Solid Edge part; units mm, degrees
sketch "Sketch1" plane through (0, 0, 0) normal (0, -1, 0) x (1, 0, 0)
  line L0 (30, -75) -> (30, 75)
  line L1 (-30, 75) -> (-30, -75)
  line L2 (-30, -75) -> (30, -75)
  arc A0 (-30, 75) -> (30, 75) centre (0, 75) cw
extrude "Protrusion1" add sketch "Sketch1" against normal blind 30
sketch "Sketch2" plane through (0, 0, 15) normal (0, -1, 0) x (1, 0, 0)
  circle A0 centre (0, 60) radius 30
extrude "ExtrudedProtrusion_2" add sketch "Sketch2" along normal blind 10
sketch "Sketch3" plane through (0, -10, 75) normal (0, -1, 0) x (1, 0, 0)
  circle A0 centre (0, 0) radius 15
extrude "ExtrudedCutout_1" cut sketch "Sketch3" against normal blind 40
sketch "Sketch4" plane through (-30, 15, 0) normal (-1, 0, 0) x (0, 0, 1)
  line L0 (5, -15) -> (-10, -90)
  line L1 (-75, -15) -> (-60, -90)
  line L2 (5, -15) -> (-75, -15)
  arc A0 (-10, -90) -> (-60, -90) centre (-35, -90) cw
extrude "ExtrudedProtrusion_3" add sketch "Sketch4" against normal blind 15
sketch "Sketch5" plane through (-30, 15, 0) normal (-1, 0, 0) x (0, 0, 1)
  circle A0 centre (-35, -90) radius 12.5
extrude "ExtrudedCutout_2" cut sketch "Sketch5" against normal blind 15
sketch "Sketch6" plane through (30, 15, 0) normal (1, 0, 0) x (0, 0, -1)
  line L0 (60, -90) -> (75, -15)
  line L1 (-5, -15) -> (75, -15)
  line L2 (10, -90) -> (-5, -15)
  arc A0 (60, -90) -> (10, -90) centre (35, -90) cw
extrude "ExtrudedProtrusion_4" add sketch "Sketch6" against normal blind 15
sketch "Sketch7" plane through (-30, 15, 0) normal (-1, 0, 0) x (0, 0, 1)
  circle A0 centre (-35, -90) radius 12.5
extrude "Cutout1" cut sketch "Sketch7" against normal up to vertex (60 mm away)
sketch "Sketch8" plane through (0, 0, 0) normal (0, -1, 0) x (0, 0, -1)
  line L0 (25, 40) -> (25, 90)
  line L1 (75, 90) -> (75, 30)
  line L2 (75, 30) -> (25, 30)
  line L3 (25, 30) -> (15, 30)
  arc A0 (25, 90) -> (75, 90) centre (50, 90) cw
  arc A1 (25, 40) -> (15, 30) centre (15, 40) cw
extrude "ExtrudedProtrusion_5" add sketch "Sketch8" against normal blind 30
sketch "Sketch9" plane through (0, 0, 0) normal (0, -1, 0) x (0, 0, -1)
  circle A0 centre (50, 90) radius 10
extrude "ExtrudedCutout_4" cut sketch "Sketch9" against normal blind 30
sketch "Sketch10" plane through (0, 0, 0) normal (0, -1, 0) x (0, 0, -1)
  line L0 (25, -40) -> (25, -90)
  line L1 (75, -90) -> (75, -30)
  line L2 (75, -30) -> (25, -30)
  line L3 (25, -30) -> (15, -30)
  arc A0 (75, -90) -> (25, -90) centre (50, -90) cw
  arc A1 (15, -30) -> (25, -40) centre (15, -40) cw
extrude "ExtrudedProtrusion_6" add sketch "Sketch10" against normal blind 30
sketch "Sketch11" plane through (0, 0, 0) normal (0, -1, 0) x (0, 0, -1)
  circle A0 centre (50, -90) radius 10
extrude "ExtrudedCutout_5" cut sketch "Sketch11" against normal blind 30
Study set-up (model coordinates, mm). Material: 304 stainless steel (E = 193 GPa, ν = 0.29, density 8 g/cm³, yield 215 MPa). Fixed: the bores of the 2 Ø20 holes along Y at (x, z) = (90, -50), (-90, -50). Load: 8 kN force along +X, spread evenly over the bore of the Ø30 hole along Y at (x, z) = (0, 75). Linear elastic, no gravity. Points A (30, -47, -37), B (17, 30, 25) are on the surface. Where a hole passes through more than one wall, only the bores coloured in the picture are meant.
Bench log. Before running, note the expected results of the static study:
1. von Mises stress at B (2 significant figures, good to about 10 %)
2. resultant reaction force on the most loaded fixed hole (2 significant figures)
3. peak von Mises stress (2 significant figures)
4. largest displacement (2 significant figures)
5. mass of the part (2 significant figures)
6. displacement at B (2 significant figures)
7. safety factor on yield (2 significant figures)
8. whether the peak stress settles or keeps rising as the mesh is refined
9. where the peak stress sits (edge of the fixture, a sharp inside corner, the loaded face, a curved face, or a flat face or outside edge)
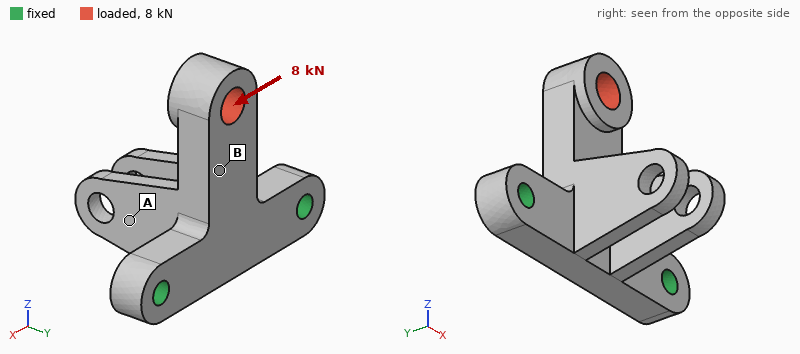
11 MPa
8.0 kN
71 MPa
74 µm
5.6 kg
22 µm
3.0
settles
a curved face
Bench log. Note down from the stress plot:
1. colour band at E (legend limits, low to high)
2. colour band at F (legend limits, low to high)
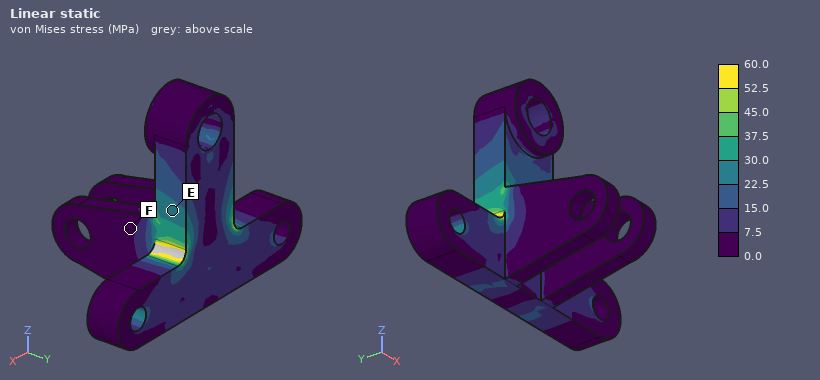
22.5 to 30.0 MPa
0.0 to 7.5 MPa
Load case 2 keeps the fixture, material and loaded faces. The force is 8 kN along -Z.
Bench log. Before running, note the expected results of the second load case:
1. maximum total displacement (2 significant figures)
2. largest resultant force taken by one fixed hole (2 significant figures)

22 µm
4.1 kN
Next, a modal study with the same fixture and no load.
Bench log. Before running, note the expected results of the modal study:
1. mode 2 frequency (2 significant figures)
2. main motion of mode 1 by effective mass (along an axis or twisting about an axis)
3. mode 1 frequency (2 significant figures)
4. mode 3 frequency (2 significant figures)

1500 Hz
along Y
790 Hz
1500 Hz
